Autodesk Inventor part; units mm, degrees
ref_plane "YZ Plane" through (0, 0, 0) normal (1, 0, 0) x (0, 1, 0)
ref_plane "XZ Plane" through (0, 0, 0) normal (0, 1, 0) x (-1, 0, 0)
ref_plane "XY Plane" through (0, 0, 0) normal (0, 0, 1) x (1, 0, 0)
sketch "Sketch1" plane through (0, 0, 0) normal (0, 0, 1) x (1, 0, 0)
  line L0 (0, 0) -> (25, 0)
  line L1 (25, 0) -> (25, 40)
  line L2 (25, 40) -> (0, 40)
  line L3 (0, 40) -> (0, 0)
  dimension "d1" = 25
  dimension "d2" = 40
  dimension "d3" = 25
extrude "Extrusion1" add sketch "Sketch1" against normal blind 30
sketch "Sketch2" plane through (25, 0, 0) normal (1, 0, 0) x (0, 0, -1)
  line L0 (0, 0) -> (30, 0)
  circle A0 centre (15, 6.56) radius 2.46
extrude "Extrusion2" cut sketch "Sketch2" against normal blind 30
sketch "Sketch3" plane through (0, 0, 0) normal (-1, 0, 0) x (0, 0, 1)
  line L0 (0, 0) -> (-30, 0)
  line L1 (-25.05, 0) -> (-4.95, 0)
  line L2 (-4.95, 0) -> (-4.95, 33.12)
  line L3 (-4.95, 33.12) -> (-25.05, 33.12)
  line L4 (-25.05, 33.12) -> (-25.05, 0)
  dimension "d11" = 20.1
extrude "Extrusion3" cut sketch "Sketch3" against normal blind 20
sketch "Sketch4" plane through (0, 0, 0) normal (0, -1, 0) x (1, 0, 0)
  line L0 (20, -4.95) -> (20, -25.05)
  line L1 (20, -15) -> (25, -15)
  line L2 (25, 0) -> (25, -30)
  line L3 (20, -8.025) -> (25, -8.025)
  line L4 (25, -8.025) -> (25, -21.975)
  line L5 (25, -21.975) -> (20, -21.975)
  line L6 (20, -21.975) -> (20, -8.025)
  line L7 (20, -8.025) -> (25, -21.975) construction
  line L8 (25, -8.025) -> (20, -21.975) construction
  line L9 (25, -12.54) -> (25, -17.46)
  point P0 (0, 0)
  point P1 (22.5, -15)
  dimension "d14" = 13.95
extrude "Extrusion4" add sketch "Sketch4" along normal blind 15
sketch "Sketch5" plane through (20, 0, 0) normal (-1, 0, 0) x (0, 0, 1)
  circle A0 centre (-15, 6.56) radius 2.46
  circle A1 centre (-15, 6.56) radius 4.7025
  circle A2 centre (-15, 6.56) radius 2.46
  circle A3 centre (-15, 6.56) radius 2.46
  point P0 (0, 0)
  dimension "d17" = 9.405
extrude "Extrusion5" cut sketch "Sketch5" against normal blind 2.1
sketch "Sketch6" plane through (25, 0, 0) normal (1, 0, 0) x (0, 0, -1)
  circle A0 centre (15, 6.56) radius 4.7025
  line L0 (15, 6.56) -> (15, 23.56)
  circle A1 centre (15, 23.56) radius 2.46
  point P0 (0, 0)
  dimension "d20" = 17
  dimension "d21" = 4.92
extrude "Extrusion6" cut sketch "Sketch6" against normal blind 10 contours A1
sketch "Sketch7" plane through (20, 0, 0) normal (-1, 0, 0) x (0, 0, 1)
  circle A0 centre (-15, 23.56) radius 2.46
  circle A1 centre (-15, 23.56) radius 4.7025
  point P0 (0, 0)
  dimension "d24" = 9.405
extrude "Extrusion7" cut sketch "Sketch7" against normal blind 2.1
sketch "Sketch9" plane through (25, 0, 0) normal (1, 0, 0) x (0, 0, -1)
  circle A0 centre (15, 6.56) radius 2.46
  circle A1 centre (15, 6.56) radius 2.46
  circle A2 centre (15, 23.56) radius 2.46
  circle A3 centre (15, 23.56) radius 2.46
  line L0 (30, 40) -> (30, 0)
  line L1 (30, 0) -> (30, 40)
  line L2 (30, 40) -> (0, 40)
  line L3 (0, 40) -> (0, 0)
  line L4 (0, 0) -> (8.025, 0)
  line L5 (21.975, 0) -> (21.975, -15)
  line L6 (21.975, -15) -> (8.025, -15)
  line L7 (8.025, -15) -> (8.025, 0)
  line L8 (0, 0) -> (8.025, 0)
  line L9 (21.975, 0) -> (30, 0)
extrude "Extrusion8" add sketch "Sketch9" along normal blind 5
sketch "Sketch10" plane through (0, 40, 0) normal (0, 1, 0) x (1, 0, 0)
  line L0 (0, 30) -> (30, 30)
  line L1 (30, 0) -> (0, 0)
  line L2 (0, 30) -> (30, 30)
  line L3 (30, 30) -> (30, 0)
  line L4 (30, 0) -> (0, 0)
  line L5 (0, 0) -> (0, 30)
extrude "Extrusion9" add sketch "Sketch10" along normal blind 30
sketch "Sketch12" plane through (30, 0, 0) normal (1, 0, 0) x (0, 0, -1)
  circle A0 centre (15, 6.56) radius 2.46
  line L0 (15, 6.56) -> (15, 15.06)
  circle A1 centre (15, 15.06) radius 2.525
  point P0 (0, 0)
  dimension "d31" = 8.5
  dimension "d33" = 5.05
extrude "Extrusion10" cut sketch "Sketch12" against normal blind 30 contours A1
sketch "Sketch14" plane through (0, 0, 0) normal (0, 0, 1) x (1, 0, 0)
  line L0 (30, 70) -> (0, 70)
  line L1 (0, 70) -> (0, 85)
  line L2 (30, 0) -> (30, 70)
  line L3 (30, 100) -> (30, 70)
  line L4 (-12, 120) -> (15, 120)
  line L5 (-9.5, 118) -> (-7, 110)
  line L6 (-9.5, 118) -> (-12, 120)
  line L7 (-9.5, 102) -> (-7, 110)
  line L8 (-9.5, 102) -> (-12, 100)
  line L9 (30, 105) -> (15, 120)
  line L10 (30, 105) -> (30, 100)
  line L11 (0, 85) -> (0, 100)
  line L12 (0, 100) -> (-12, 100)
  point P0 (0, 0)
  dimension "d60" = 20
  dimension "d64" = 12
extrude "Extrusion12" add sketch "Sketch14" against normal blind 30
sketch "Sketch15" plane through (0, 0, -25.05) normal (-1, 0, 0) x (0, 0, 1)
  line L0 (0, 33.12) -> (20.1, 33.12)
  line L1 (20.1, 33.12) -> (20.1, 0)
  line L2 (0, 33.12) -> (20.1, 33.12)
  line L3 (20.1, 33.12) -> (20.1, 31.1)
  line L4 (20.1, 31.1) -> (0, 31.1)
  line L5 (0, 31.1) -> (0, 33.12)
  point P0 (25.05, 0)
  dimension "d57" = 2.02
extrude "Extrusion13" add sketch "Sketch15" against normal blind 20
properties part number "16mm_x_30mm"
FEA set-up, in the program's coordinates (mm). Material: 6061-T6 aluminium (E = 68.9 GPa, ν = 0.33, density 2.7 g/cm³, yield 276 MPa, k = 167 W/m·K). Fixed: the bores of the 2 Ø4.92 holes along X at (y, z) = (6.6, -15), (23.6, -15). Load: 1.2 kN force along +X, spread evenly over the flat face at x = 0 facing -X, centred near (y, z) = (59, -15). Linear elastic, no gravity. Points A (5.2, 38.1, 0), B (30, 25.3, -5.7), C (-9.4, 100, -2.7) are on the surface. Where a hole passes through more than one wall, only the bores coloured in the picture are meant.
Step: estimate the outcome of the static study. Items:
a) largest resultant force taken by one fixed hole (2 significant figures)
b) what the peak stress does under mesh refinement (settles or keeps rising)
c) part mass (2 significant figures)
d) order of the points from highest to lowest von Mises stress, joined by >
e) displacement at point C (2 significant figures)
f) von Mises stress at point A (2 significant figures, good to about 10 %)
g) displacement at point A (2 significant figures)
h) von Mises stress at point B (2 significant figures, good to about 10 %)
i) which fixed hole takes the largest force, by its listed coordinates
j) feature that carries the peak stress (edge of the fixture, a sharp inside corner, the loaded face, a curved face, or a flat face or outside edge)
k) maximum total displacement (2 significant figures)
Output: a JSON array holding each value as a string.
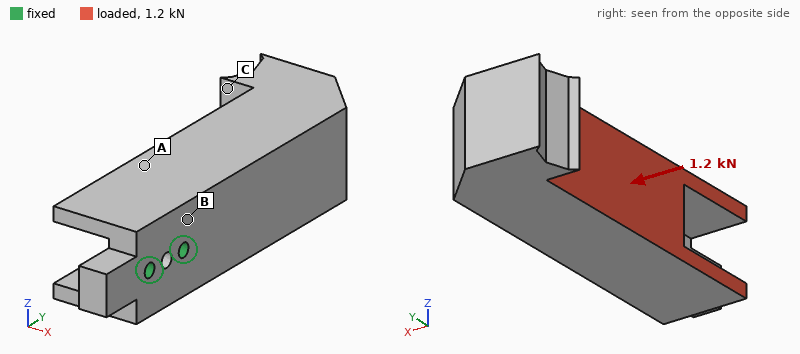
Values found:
["2.8 kN", "keeps rising", "270 g", "B > A > C", "0.095 mm", "11 MPa", "0.026 mm", "18 MPa", "(23.6, -15)", "edge of the fixture", "0.12 mm"]
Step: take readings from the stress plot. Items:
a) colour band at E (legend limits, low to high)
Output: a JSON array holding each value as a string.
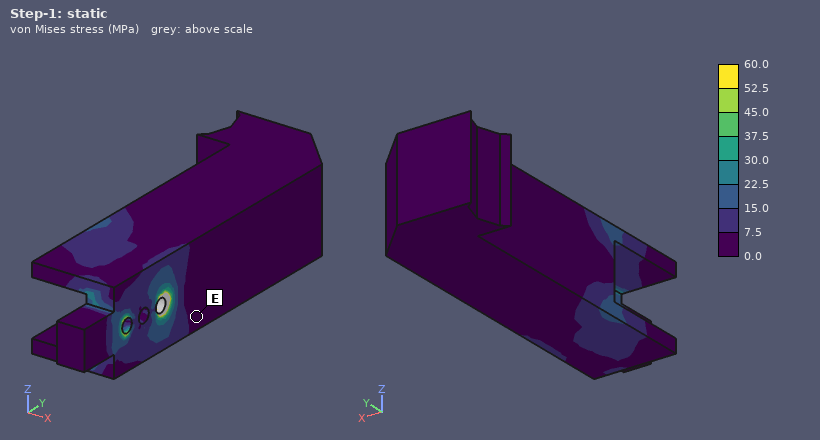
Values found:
["0.0 to 7.5 MPa"]
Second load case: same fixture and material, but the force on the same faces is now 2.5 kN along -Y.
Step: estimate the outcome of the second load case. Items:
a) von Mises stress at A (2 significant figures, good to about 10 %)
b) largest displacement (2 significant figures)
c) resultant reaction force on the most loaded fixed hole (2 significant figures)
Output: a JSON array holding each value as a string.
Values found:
["16 MPa", "0.16 mm", "2.9 kN"]
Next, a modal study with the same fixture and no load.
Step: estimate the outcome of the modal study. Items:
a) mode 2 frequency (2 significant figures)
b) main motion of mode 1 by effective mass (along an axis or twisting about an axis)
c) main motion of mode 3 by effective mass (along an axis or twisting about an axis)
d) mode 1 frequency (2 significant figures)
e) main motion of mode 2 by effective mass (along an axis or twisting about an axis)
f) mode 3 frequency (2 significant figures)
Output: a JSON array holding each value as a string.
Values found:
["1300 Hz", "along X", "twisting about Y", "1100 Hz", "along Z", "3300 Hz"]
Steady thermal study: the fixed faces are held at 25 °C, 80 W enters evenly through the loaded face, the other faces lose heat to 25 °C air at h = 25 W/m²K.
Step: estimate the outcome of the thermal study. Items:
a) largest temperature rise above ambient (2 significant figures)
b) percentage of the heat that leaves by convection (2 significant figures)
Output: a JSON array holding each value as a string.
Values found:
["32 K", "10 %"]
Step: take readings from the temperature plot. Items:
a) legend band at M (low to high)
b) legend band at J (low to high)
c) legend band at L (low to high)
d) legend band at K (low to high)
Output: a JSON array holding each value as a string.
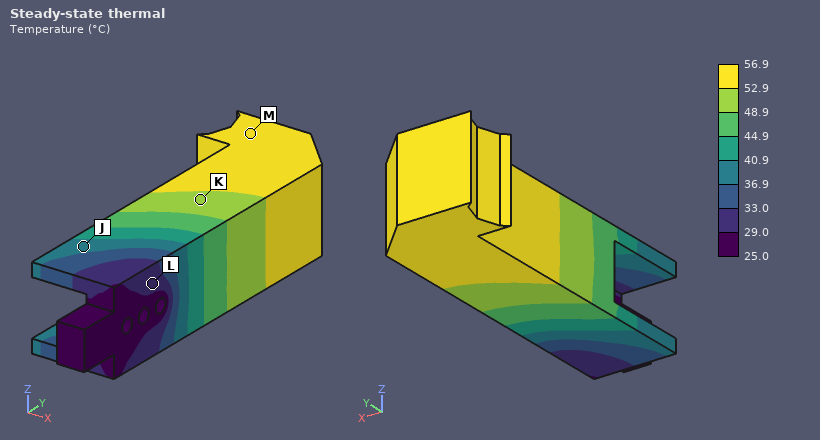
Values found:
["52.9 to 56.9 °C", "36.9 to 40.9 °C", "29.0 to 33.0 °C", "48.9 to 52.9 °C"]
